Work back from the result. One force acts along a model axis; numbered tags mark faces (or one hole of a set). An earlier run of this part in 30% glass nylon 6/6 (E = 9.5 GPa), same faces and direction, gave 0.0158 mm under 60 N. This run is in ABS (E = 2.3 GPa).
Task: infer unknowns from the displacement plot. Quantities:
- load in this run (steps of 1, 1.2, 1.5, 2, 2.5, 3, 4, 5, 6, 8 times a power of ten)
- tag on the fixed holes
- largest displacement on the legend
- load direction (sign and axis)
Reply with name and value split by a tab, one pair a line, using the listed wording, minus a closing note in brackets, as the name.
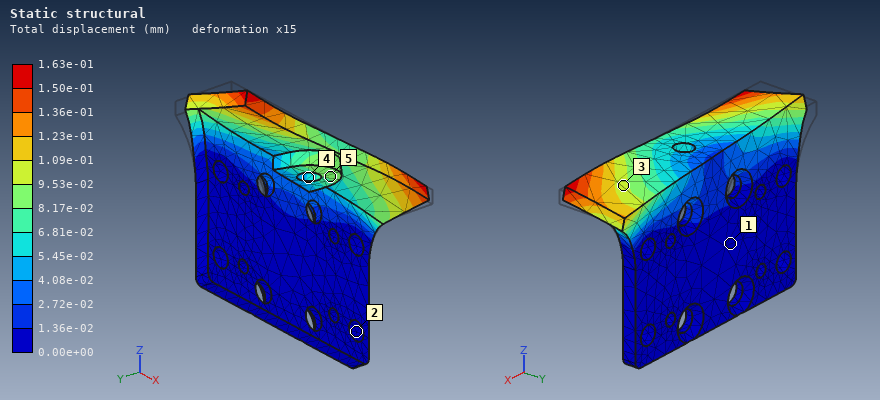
load in this run	150 N
tag on the fixed holes	2
largest displacement on the legend	1.63e-01 mm
load direction	+X
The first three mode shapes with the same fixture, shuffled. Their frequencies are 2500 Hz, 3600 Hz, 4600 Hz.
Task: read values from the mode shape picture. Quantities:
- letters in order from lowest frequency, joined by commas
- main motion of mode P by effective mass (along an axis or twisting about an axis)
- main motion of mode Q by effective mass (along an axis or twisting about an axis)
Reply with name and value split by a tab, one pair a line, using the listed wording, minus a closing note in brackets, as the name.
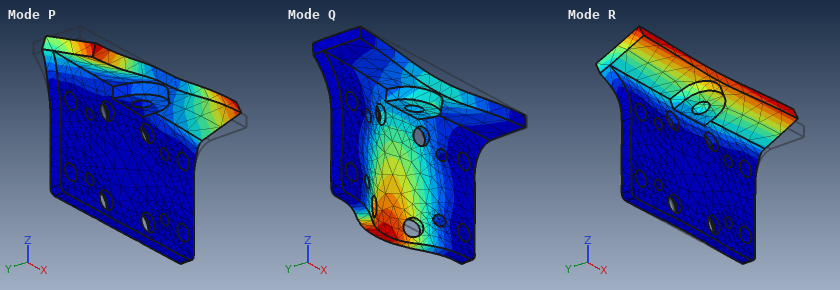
letters in order from lowest frequency, joined by commas	R, P, Q
main motion of mode P by effective mass	twisting about Z
main motion of mode Q by effective mass	along Y
